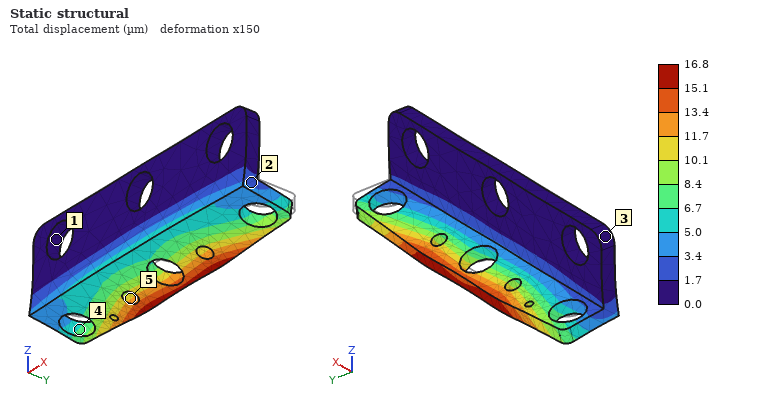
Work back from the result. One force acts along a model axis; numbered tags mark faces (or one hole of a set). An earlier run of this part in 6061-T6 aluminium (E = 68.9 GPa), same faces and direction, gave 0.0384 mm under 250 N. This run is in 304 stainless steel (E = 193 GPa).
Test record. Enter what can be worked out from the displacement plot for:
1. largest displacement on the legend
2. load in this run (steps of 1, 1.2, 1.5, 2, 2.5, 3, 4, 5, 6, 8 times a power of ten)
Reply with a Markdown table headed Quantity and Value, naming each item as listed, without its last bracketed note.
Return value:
| Quantity | Value |
|---|---|
| largest displacement on the legend | 16.8 µm |
| load in this run | 300 N |
